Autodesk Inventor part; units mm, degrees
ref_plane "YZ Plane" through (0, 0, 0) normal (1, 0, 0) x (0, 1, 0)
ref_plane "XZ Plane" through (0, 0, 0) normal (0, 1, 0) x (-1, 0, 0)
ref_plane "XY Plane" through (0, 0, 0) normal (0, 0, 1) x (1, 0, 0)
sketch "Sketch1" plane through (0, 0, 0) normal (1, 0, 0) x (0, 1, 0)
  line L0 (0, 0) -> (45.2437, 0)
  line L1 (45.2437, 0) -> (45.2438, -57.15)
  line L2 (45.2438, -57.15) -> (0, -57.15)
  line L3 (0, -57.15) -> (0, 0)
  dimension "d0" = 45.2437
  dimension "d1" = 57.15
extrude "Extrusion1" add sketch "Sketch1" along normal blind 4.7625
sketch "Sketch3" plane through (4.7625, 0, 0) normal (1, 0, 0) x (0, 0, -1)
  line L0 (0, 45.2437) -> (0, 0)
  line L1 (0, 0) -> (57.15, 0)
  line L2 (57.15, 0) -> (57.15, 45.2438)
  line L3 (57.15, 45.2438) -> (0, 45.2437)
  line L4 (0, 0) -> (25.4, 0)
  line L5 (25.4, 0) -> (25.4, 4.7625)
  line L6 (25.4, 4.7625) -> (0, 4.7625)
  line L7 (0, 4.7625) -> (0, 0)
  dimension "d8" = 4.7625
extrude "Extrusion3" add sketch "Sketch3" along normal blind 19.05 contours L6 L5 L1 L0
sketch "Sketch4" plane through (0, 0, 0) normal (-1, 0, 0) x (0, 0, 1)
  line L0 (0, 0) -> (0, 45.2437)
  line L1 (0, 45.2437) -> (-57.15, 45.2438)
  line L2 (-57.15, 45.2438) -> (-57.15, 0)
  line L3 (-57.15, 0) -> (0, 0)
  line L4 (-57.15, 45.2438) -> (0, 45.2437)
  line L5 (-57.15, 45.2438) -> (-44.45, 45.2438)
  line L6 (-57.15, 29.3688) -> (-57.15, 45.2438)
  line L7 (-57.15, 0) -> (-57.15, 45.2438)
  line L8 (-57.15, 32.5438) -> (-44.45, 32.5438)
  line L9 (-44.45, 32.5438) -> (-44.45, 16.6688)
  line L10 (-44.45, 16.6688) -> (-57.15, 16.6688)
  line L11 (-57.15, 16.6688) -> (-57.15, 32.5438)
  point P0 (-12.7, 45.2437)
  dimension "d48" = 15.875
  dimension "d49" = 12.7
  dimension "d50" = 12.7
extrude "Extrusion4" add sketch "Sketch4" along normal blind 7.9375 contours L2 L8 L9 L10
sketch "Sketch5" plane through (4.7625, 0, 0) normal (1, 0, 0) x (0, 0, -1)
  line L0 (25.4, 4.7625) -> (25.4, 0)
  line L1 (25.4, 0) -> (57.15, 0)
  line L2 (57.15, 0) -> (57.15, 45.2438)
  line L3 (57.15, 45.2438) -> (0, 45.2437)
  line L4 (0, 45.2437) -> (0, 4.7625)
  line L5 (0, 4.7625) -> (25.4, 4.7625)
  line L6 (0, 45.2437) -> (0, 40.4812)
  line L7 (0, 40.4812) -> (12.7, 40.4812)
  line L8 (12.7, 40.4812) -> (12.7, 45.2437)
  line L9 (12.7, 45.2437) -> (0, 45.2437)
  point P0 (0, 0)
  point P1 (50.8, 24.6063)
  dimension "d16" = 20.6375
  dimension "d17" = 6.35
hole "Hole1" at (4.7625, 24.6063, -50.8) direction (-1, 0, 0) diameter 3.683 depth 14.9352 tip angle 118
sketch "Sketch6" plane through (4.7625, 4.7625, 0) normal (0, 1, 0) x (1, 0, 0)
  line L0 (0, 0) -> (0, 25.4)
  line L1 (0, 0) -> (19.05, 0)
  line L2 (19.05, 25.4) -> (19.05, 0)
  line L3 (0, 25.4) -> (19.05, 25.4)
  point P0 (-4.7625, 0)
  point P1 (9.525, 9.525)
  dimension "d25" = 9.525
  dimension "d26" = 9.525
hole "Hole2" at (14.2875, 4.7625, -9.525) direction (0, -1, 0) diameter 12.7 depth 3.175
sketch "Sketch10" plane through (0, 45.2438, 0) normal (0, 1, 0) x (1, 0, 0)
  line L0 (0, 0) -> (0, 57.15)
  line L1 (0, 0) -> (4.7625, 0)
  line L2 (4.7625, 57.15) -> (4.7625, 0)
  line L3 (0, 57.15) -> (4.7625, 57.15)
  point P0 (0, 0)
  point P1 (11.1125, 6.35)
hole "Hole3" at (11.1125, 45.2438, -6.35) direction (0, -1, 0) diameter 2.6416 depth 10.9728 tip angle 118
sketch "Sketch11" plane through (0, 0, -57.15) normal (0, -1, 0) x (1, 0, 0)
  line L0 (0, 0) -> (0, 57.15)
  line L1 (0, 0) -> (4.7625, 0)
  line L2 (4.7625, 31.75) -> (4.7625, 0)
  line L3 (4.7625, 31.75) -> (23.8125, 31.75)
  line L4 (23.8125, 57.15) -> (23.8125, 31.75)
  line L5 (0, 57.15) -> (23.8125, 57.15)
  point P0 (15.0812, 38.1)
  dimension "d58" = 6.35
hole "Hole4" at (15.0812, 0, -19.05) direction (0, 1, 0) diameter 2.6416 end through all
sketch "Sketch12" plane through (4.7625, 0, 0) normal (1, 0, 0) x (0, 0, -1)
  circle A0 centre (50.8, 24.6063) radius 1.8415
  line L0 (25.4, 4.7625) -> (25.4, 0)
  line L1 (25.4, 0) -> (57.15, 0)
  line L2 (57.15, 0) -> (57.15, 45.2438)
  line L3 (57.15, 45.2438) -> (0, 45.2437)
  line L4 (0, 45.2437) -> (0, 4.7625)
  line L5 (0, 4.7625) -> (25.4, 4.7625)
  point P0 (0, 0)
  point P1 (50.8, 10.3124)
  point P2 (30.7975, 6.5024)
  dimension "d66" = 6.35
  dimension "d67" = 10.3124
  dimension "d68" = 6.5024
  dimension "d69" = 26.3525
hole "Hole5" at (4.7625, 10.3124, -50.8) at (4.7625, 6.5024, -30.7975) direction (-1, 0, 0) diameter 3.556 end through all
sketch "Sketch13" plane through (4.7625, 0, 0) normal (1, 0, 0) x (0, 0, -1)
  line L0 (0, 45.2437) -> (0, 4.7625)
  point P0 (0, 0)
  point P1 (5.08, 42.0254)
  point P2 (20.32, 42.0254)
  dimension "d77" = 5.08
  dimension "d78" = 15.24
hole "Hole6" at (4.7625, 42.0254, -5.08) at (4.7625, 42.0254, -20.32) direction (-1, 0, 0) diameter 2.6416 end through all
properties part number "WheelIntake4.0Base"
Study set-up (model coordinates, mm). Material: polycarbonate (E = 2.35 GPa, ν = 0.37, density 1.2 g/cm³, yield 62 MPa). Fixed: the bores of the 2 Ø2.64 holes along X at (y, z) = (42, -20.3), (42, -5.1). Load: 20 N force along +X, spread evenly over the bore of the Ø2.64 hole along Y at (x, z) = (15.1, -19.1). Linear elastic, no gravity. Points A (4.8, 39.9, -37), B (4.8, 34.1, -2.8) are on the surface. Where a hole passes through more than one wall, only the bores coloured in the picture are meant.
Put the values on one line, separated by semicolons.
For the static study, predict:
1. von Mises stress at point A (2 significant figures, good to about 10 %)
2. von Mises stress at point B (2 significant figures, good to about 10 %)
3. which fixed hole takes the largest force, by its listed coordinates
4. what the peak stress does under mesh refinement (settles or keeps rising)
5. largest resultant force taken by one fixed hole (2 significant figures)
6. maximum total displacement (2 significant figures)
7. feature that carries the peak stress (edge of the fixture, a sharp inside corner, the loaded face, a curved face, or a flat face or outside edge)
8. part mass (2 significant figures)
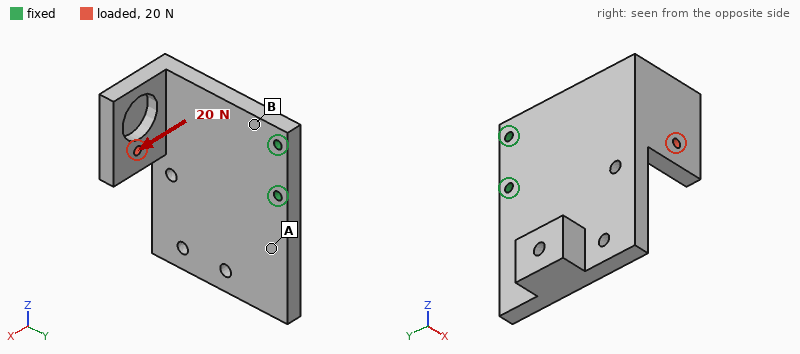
2.0 MPa; 4.8 MPa; (42, -20.3); keeps rising; 18 N; 0.79 mm; edge of the fixture; 19 g
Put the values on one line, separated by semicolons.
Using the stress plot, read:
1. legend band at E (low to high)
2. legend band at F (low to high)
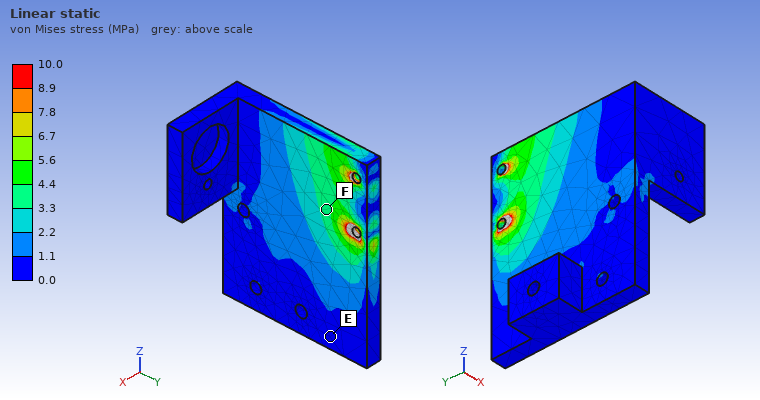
0.0 to 1.1 MPa; 3.3 to 4.4 MPa
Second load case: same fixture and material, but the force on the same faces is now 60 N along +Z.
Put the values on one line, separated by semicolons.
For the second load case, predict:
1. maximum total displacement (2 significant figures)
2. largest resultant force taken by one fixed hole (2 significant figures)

0.74 mm; 150 N
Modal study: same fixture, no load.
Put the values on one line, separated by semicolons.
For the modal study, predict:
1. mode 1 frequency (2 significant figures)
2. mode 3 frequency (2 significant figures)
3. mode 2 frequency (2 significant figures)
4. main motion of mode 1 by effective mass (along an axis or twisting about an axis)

320 Hz; 980 Hz; 480 Hz; along X
